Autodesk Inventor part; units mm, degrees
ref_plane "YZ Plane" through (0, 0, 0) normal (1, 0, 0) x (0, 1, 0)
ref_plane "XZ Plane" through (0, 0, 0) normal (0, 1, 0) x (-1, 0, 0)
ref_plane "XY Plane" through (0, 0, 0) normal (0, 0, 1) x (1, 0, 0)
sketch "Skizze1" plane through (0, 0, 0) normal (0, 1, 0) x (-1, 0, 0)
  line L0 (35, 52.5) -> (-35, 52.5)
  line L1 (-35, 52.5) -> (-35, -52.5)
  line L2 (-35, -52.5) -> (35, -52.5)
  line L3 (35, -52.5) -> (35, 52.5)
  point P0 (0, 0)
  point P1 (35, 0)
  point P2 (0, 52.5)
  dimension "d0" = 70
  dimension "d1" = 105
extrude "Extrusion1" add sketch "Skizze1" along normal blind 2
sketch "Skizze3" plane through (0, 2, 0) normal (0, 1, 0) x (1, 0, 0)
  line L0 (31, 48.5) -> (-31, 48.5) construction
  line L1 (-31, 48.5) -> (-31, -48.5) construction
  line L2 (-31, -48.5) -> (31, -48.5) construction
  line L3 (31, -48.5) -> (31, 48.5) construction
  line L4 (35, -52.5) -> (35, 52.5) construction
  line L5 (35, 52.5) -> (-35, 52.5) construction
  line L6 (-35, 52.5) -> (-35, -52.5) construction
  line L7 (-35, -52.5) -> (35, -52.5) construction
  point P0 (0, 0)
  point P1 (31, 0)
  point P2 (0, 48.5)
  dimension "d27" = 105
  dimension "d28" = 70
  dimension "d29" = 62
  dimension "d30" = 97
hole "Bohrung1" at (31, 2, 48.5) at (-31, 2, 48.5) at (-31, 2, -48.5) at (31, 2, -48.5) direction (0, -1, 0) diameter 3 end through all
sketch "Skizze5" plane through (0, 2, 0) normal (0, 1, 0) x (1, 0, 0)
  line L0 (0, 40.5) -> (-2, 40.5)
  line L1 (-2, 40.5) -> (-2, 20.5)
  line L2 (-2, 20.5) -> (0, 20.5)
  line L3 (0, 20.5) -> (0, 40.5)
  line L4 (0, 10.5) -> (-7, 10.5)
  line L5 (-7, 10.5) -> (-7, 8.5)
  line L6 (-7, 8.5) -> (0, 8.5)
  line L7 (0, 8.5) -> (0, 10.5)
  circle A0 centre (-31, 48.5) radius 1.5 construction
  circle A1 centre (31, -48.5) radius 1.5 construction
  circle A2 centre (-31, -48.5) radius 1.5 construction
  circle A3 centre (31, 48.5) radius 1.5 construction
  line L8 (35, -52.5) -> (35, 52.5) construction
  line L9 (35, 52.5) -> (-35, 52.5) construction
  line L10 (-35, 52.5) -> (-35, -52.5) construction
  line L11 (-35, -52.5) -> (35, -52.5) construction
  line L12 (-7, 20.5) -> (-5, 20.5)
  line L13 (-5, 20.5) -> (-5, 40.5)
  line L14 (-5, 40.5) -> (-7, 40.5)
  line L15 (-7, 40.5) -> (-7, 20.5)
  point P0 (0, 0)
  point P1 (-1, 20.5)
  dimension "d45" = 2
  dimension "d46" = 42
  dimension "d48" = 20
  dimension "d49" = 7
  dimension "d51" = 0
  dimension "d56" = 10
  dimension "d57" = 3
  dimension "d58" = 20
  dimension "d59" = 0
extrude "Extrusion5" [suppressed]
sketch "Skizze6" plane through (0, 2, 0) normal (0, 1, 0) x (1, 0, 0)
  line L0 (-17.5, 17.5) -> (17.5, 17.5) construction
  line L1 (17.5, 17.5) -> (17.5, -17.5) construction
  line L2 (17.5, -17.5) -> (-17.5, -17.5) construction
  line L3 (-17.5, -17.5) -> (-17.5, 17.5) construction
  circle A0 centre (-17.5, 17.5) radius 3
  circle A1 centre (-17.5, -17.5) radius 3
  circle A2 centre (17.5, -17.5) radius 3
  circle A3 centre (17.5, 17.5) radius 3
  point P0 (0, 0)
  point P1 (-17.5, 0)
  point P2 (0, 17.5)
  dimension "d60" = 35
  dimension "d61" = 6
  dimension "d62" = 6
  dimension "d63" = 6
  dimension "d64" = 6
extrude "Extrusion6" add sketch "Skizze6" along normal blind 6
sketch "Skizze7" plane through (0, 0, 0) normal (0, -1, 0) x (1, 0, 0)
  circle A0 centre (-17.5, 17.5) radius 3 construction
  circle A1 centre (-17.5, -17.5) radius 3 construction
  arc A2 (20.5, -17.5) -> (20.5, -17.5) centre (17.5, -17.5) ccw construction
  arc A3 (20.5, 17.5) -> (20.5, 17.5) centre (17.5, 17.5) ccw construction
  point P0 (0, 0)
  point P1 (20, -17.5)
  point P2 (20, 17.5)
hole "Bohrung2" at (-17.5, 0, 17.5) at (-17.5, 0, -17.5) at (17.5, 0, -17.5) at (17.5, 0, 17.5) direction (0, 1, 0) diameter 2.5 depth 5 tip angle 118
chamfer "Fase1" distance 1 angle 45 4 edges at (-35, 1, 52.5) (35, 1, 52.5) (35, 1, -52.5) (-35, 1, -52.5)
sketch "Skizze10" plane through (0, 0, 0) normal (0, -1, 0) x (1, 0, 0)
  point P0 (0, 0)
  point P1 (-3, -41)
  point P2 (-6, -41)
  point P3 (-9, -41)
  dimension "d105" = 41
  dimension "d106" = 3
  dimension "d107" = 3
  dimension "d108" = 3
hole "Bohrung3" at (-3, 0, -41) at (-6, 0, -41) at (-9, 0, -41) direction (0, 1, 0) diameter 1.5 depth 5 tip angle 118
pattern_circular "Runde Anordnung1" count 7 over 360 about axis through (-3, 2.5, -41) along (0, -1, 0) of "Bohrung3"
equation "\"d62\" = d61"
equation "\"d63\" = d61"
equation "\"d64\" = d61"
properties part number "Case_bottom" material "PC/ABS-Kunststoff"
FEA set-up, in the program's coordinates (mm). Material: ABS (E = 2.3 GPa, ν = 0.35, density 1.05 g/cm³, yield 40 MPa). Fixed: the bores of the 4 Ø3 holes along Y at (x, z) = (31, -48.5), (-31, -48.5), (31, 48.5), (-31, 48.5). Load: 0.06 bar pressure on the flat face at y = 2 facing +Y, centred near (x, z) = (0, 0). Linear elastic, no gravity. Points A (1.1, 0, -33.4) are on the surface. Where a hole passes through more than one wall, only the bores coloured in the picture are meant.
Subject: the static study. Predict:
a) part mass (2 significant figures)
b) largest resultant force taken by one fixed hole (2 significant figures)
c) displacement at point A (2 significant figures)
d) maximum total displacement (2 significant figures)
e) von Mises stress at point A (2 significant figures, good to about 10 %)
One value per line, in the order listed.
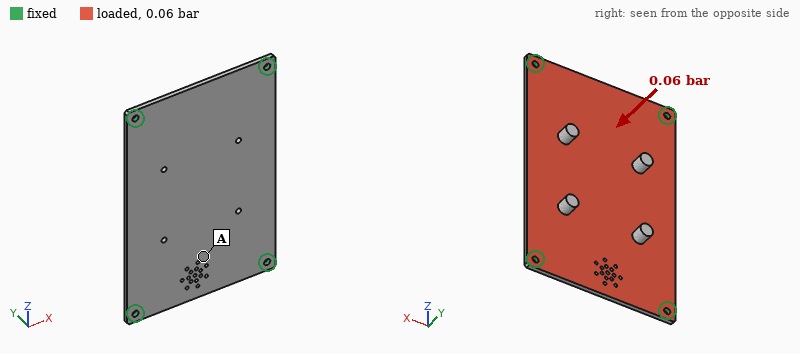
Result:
16 g
11 N
0.71 mm
1.4 mm
2.1 MPa
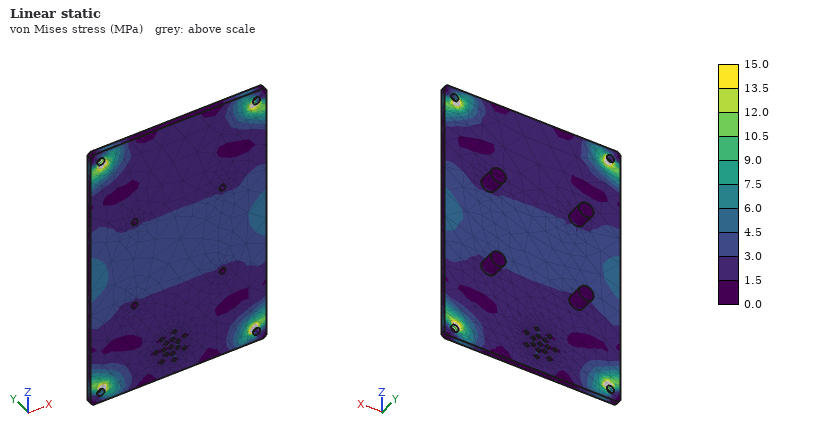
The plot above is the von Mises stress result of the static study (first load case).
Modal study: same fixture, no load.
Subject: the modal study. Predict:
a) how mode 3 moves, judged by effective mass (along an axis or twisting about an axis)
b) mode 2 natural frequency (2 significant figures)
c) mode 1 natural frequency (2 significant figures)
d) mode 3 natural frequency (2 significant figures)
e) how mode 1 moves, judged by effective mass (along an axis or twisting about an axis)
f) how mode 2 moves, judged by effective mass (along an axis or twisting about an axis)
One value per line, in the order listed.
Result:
twisting about X
430 Hz
250 Hz
640 Hz
along Y
twisting about Z
